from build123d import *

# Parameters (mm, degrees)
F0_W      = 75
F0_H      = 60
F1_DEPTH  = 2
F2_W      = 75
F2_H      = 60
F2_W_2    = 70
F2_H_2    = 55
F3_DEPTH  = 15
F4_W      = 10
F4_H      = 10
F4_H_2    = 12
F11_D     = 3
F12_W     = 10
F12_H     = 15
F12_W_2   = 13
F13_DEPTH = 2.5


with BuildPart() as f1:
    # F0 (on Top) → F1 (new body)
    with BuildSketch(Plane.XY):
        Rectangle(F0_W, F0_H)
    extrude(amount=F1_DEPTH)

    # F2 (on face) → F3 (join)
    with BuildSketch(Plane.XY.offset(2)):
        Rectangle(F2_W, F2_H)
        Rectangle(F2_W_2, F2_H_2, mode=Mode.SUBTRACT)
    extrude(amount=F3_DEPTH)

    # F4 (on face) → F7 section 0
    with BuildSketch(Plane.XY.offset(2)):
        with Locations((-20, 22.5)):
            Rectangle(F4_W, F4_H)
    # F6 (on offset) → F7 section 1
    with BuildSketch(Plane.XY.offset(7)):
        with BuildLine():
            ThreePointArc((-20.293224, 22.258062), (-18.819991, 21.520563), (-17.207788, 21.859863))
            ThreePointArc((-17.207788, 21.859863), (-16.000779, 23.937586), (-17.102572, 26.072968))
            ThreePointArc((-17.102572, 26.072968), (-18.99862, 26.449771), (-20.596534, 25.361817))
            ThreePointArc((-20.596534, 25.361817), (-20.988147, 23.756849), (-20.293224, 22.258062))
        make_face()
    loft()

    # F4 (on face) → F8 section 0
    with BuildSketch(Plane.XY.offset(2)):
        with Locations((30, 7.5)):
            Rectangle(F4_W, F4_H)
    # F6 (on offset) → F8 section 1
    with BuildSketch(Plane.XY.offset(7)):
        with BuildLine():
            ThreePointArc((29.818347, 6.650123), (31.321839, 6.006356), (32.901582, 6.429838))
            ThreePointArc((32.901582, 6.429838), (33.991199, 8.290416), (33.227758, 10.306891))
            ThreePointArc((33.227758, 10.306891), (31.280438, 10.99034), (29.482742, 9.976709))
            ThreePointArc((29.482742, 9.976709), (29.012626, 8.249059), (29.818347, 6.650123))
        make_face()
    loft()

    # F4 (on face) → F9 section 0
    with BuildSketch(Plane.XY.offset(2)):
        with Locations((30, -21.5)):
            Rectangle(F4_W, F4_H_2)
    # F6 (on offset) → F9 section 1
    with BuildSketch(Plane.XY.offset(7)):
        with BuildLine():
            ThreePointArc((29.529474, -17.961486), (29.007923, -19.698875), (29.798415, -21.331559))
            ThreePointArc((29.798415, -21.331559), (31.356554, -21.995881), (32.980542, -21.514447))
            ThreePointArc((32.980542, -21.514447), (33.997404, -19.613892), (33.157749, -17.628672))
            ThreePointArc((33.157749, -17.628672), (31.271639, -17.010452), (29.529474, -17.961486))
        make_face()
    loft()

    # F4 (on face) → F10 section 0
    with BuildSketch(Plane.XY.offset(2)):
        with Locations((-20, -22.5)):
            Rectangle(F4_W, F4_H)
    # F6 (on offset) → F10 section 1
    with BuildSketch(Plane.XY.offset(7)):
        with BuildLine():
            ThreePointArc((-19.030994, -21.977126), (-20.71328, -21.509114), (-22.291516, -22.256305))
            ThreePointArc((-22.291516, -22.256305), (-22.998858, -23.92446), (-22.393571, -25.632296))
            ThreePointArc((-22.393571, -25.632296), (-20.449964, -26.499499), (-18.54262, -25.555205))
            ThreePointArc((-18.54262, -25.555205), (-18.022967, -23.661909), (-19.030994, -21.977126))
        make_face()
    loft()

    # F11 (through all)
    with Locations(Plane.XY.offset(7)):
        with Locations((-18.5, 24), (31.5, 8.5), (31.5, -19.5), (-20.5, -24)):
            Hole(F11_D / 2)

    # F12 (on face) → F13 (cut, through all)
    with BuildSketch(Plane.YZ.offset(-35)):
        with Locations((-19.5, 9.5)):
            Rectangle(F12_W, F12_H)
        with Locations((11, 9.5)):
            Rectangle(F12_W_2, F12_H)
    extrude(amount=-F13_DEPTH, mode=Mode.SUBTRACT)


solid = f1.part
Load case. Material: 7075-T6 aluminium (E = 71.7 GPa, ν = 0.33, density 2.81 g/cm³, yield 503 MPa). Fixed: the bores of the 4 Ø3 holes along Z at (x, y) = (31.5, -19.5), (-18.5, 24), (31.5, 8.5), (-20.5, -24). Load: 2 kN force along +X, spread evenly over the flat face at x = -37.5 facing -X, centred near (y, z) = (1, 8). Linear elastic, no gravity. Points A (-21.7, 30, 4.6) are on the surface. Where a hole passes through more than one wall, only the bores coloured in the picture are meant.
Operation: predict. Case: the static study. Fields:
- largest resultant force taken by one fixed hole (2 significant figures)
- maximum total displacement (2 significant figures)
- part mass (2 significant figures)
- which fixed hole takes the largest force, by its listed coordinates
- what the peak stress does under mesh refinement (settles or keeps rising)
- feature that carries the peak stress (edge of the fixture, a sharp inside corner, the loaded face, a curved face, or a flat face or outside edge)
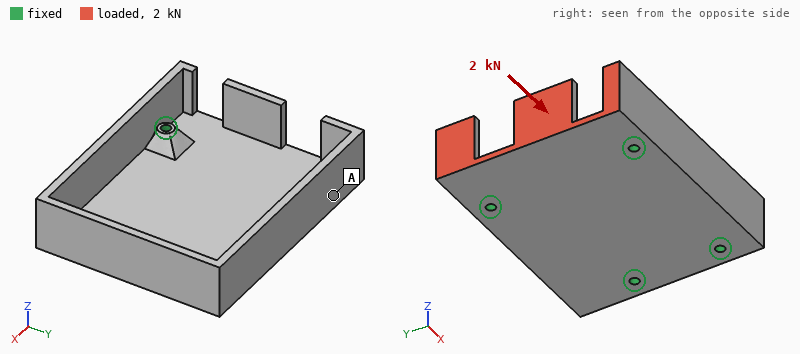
790 N
0.96 mm
53 g
(-18.5, 24)
keeps rising
a sharp inside corner
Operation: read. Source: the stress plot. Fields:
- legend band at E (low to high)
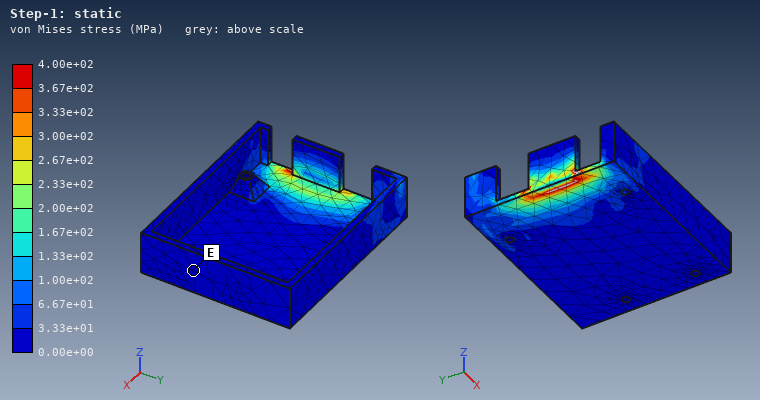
0.00e+00 to 3.33e+01 MPa
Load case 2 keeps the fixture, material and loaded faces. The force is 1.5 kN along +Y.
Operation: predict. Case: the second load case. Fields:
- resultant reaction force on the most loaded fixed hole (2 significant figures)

960 N
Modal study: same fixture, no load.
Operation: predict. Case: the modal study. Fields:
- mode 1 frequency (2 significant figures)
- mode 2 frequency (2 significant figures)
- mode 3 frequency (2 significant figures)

3300 Hz
4700 Hz
4900 Hz
